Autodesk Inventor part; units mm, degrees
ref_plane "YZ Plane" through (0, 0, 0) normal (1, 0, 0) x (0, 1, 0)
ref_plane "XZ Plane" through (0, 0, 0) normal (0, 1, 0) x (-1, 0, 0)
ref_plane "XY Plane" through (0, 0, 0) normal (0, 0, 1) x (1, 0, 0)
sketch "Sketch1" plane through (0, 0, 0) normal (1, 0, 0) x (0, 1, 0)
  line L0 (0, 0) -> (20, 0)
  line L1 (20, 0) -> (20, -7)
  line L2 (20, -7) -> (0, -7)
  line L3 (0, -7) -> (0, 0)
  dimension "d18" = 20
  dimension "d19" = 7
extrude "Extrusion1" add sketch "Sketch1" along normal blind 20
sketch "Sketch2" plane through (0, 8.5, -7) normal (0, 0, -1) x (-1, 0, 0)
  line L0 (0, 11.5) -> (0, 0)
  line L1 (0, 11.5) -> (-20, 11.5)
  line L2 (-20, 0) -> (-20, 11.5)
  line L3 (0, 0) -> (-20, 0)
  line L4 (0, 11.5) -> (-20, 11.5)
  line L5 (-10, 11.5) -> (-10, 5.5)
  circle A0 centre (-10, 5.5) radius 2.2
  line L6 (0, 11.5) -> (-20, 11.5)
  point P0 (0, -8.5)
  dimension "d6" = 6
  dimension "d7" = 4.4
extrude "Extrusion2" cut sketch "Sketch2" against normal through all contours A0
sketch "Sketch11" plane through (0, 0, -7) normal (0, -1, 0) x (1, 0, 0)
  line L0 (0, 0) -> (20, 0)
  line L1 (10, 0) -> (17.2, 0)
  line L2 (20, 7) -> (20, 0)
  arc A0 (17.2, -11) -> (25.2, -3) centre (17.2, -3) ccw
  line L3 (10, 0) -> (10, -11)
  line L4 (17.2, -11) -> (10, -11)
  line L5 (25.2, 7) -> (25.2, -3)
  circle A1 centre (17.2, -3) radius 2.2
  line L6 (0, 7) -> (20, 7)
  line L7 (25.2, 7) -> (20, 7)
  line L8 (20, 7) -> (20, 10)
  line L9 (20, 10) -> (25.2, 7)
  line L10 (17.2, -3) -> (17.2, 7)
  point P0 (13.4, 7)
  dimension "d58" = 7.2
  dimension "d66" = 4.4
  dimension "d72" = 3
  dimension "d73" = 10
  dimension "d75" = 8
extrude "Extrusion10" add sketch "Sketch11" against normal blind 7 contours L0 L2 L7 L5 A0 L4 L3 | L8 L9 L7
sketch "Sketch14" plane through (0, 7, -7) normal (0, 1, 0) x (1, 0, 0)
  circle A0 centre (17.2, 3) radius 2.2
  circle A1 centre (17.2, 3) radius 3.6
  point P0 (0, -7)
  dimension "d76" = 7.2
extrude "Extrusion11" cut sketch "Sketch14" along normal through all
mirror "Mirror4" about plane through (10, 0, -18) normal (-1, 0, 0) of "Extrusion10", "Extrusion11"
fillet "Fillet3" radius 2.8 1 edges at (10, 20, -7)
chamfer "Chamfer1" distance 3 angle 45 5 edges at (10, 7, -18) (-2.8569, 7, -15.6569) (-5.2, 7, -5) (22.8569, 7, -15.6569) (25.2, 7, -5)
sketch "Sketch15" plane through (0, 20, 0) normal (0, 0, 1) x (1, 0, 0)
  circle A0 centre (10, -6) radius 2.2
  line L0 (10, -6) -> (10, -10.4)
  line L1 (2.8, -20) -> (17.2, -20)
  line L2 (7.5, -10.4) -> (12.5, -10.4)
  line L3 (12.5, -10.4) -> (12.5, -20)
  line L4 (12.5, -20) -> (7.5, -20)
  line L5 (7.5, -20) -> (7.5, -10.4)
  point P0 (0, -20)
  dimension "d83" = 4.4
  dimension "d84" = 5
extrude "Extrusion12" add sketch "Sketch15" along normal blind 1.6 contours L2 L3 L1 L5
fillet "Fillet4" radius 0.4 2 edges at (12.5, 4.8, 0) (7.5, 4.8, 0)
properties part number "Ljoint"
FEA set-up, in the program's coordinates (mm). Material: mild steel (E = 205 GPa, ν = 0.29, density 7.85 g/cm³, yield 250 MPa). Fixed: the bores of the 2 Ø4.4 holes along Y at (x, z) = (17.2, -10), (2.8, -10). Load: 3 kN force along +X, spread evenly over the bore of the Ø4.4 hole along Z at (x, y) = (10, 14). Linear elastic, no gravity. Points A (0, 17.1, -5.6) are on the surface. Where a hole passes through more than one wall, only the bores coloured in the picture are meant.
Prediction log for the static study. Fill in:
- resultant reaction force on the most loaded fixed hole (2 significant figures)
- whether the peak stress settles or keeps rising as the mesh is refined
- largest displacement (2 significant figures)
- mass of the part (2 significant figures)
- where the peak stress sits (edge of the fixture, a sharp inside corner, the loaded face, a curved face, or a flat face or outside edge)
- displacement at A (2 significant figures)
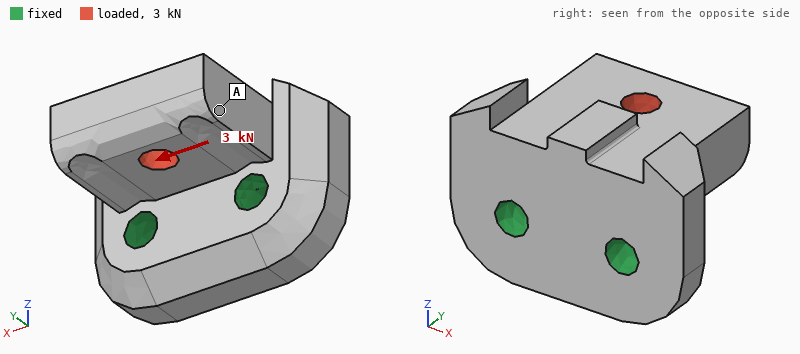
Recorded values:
2.4 kN
keeps rising
10 µm
39 g
edge of the fixture
9.3 µm
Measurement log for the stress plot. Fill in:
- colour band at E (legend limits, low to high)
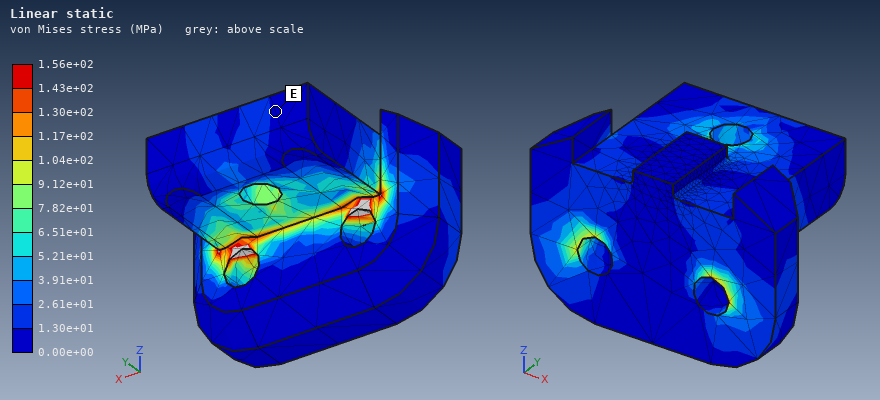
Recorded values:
0.00e+00 to 1.30e+01 MPa
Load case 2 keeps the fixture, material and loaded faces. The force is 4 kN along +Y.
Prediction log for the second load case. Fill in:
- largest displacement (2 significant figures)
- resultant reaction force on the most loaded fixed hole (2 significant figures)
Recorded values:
13 µm
2.0 kN
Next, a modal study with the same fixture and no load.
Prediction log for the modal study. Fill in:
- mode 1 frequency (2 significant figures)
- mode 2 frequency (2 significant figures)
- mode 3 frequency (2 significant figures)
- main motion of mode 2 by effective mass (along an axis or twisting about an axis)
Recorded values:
16 kHz
26 kHz
34 kHz
along X
